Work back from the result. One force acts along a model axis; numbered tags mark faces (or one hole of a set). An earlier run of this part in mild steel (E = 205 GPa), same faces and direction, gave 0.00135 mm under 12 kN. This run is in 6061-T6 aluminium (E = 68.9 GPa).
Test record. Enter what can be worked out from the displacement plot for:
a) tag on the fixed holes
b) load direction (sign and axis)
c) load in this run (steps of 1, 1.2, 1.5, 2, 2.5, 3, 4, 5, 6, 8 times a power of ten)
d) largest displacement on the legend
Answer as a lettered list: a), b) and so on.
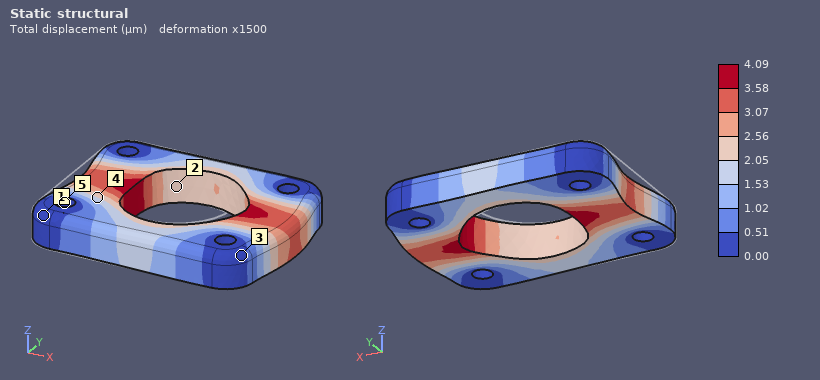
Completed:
a) 5
b) +X
c) 12 kN
d) 4.09 µm
